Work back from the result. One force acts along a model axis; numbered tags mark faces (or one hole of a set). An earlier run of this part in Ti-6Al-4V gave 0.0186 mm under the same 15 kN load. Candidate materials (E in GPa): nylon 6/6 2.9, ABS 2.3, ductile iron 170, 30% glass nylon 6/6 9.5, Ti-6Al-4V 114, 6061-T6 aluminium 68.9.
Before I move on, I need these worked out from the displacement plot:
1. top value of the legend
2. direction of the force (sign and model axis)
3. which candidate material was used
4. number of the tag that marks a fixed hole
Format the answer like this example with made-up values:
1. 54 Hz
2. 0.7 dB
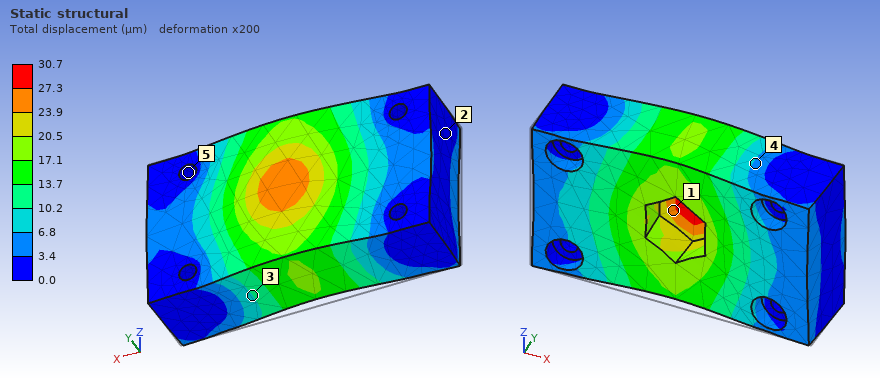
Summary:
1. 30.7 µm
2. +Y
3. 6061-T6 aluminium
4. 5
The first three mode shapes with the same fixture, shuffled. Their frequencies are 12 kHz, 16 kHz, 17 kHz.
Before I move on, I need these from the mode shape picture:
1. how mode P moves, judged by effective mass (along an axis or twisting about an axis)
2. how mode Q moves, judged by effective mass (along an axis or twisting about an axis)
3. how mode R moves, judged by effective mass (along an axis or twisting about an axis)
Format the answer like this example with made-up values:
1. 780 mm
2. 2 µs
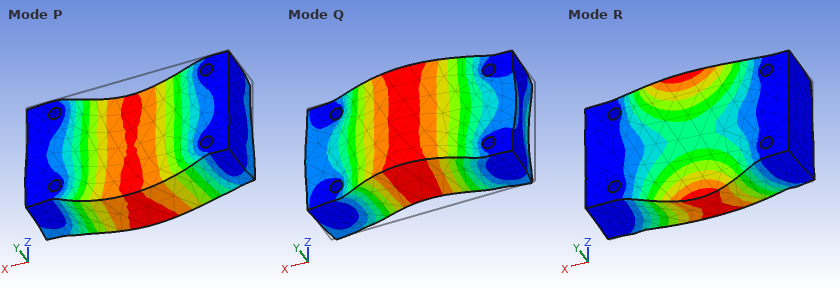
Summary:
1. along Z
2. along Y
3. twisting about X
